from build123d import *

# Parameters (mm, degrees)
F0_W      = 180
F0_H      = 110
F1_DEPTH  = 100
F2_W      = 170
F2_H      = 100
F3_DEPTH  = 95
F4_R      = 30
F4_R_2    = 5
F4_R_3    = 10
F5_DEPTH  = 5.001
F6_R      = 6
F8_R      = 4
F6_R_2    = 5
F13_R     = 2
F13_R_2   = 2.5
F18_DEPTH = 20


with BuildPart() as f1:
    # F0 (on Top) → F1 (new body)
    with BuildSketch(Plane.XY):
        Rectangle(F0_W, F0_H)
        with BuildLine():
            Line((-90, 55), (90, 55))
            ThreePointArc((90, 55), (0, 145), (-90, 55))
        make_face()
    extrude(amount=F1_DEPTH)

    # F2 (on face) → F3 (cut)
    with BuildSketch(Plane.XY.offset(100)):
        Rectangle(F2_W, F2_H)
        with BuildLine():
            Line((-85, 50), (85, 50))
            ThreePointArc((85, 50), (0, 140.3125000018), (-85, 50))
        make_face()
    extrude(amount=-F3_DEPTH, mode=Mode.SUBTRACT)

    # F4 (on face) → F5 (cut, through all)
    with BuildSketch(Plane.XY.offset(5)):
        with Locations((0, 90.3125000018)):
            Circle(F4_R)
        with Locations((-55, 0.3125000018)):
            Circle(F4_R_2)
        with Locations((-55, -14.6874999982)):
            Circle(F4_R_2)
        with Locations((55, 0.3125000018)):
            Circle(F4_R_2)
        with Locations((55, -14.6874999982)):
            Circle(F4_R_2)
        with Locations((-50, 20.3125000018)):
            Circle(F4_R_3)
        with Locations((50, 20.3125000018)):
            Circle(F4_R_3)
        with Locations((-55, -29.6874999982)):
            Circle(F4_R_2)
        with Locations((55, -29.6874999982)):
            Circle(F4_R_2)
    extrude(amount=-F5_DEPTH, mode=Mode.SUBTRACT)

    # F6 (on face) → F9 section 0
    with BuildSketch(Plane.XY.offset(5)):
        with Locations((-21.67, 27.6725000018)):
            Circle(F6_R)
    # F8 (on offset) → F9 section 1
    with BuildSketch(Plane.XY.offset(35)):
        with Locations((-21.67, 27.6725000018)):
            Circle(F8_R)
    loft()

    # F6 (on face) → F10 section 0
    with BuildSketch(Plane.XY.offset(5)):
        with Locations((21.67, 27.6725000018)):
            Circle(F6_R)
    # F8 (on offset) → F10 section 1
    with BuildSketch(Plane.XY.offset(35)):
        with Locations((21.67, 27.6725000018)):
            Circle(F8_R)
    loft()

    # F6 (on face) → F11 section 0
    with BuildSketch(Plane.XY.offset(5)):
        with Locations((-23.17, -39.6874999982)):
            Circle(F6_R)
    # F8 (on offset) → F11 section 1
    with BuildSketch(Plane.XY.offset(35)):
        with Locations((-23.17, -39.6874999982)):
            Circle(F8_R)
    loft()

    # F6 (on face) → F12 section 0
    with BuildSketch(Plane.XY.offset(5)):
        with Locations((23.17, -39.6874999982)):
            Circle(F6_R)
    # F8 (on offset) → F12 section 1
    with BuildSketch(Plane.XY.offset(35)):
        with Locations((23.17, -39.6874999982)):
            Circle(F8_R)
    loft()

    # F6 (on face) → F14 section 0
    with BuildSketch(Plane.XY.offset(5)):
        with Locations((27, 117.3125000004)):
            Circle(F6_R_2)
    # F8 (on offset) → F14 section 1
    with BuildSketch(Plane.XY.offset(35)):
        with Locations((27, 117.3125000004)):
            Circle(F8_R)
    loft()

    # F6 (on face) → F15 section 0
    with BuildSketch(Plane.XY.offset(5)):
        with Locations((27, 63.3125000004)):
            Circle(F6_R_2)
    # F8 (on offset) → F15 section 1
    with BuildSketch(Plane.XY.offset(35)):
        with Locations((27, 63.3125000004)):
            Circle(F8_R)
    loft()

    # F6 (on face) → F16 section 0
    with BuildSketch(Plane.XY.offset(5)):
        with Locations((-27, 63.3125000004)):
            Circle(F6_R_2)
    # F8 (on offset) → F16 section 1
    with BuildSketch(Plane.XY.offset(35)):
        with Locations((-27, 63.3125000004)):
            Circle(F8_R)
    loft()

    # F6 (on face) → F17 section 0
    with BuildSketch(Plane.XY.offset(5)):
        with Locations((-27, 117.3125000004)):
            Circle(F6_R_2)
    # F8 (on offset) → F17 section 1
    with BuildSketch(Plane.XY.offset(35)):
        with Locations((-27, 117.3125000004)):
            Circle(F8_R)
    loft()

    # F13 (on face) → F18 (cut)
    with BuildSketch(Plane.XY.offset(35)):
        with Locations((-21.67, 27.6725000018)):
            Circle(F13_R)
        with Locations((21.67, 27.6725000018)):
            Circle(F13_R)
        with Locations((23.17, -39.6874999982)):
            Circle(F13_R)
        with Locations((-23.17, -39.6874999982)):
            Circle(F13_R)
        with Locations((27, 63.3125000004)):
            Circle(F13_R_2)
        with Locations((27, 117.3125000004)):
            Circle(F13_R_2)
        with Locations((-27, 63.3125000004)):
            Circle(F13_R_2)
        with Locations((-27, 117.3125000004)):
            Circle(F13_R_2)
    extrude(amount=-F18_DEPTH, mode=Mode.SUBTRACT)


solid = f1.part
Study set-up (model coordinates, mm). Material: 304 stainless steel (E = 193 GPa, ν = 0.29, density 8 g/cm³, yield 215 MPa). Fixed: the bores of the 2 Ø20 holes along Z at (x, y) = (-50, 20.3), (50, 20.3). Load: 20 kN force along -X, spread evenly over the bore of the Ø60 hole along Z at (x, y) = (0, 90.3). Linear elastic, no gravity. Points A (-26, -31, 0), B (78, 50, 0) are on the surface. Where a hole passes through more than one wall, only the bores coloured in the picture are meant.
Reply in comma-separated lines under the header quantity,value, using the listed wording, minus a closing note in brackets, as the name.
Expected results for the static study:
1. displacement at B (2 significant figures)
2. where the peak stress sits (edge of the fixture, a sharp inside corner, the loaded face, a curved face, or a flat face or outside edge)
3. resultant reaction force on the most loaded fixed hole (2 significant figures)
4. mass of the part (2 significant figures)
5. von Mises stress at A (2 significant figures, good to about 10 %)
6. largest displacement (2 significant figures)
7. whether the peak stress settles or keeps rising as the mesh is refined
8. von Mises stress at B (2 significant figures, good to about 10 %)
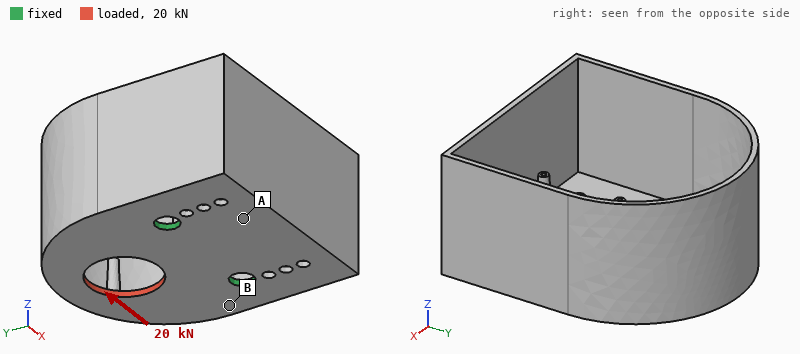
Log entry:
quantity,value
displacement at B,21 µm
where the peak stress sits,edge of the fixture
resultant reaction force on the most loaded fixed hole,15 kN
mass of the part,3.7 kg
von Mises stress at A,11 MPa
largest displacement,70 µm
whether the peak stress settles or keeps rising as the mesh is refined,keeps rising
von Mises stress at B,25 MPa
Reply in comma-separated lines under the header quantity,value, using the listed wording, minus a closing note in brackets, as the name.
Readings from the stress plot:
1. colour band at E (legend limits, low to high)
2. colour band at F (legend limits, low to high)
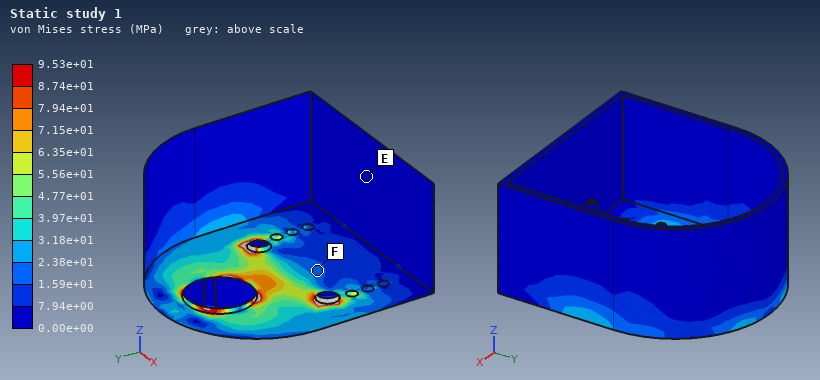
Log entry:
quantity,value
colour band at E,0.00e+00 to 7.94e+00 MPa
colour band at F,1.59e+01 to 2.38e+01 MPa
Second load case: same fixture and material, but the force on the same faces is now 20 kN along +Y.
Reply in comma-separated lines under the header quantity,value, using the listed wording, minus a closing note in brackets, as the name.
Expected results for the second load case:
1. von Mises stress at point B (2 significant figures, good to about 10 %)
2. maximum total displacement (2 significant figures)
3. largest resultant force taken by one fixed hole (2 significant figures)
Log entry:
quantity,value
von Mises stress at point B,11 MPa
maximum total displacement,29 µm
largest resultant force taken by one fixed hole,10 kN
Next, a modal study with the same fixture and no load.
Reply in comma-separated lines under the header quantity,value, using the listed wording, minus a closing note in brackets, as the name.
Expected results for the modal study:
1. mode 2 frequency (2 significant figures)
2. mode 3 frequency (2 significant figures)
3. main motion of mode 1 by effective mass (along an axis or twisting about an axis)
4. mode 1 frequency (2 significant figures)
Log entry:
quantity,value
mode 2 frequency,370 Hz
mode 3 frequency,580 Hz
main motion of mode 1 by effective mass,along Y
mode 1 frequency,210 Hz
